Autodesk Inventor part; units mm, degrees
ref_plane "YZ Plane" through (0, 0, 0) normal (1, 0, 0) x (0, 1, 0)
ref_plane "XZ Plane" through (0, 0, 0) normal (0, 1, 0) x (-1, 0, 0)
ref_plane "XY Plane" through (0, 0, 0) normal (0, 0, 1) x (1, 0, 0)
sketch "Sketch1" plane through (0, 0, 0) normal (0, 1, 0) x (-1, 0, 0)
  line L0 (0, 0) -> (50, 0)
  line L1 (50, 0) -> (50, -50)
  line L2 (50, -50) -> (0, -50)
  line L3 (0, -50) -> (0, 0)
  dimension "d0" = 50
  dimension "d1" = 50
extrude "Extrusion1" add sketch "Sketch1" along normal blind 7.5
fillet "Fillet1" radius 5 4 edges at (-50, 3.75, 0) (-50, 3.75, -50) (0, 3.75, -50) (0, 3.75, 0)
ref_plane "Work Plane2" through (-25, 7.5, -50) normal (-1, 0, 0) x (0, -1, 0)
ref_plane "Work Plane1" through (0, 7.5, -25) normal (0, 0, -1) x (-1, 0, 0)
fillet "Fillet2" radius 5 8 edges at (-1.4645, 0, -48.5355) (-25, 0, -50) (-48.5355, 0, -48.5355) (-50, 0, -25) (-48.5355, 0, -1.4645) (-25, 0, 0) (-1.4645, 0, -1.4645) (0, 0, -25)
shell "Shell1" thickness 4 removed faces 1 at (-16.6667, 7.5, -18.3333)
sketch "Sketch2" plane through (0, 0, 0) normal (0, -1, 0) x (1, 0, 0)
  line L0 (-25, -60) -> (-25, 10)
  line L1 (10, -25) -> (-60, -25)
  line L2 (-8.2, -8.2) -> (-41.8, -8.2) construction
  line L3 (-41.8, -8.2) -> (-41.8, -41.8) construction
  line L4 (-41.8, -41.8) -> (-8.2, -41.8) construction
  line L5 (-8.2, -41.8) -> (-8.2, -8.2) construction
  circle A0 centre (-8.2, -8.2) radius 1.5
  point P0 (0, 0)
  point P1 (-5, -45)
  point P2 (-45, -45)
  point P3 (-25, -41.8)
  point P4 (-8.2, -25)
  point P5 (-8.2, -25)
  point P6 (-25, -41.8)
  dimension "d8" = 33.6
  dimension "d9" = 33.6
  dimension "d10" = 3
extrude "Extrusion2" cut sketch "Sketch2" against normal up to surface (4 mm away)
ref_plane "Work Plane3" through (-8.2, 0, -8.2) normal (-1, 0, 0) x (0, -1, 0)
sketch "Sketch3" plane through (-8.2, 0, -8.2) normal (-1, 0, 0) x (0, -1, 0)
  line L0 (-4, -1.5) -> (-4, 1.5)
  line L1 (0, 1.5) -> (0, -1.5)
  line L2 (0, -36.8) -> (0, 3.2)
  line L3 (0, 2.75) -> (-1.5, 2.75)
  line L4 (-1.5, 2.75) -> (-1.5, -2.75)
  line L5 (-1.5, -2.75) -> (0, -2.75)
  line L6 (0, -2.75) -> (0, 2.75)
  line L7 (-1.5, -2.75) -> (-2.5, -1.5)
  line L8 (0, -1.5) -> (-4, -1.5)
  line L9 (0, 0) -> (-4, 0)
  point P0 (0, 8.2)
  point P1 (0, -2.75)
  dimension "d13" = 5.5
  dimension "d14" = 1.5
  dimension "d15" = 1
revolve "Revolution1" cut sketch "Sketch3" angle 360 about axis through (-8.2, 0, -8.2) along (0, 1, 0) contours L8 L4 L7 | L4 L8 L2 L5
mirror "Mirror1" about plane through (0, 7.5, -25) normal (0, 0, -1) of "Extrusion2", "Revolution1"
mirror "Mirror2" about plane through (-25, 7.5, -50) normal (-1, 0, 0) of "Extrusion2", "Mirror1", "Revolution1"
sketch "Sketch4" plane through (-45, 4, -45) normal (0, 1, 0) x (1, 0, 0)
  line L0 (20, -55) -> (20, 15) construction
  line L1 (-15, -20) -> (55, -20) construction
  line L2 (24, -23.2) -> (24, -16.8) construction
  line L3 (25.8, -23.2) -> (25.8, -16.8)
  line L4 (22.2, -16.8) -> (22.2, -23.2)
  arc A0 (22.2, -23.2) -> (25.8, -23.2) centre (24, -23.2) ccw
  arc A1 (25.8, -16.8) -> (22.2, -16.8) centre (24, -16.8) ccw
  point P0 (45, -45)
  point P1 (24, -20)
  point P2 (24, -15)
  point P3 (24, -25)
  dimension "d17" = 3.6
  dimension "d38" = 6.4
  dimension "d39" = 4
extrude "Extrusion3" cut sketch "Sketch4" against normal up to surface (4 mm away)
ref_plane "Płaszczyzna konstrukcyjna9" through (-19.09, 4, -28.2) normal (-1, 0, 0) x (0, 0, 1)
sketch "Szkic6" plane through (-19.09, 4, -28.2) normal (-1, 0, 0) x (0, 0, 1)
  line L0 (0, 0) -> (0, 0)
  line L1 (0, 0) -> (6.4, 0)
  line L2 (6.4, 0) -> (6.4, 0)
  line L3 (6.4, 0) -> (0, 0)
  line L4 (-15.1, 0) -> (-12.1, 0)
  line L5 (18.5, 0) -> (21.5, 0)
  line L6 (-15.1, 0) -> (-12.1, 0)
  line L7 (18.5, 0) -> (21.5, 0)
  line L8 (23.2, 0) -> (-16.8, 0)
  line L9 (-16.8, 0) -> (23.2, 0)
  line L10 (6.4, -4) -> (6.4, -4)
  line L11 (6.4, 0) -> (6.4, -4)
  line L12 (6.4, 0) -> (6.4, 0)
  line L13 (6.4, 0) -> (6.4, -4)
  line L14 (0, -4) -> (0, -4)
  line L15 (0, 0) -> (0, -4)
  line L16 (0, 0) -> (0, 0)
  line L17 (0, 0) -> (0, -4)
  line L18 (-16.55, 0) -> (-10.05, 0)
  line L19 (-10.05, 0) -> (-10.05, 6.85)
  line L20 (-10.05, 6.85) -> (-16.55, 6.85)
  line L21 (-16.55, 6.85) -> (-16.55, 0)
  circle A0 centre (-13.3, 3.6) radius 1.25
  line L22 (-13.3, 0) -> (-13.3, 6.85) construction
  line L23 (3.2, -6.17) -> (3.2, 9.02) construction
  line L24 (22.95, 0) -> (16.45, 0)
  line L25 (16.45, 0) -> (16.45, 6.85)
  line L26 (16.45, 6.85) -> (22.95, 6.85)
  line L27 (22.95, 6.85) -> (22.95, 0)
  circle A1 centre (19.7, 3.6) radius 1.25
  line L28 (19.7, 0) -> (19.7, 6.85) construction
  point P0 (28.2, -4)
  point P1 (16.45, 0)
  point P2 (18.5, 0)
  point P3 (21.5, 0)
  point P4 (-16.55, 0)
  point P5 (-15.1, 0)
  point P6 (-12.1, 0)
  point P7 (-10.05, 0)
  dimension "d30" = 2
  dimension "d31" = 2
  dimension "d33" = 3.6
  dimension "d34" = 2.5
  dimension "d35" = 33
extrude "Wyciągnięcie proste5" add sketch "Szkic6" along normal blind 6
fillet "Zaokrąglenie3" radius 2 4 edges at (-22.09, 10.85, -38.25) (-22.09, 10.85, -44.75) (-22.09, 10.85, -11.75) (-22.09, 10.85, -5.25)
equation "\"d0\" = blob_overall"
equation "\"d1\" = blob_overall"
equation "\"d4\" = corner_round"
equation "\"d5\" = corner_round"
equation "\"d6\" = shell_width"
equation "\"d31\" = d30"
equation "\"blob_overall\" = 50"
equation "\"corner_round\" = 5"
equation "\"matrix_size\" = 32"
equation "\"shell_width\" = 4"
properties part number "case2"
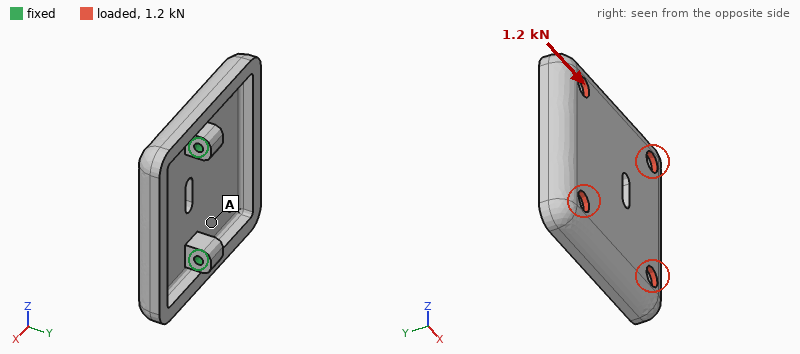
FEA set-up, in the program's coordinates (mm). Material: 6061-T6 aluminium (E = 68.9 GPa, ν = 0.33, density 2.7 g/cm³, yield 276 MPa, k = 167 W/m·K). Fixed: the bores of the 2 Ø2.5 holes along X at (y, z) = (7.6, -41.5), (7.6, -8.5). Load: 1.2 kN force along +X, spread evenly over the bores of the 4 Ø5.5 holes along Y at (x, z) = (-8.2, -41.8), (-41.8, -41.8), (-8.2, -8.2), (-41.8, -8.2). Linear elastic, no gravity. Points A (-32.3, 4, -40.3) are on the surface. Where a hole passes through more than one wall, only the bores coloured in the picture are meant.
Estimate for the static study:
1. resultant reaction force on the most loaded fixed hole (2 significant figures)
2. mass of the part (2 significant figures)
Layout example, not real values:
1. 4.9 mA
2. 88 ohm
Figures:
1. 600 N
2. 31 g
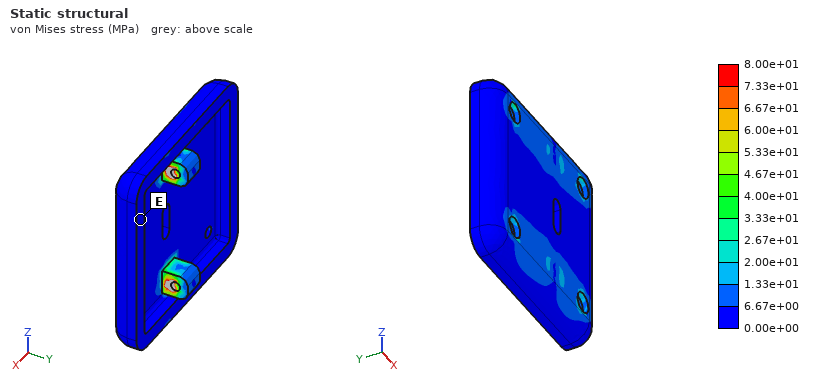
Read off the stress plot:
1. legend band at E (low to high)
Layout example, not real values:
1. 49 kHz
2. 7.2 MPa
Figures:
1. 0.00e+00 to 6.67e+00 MPa
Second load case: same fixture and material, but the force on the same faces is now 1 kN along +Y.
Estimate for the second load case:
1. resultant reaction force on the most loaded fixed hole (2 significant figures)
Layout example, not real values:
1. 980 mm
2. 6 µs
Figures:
1. 510 N
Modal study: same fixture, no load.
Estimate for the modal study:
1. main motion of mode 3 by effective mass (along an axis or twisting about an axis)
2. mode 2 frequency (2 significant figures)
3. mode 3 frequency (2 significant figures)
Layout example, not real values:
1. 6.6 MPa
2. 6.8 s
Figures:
1. along Y
2. 5700 Hz
3. 6200 Hz
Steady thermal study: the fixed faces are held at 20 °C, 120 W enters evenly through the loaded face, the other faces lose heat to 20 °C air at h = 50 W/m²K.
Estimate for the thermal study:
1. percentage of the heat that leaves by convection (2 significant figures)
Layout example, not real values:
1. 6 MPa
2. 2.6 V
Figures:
1. 14 %
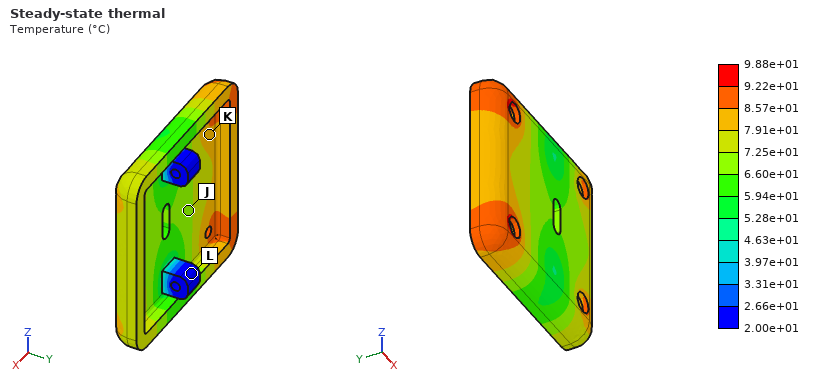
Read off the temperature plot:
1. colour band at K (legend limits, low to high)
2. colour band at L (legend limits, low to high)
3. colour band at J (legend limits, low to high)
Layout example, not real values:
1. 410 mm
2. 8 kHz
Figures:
1. 7.91e+01 to 8.57e+01 °C
2. 2.00e+01 to 2.66e+01 °C
3. 6.60e+01 to 7.25e+01 °C
